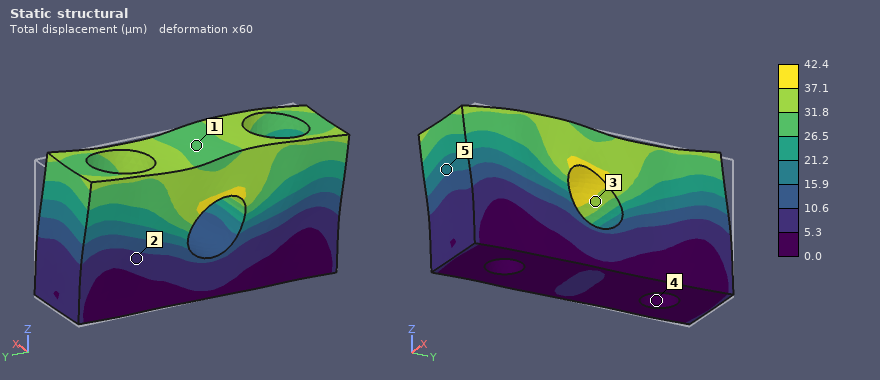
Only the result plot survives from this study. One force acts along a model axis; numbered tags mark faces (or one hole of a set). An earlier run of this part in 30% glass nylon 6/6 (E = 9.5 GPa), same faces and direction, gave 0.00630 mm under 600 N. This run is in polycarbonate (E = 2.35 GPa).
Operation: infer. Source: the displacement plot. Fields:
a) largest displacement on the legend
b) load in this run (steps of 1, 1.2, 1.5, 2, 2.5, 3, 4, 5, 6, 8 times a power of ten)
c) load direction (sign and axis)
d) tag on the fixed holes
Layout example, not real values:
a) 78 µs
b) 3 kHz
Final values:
a) 42.4 µm
b) 1 kN
c) -Y
d) 4
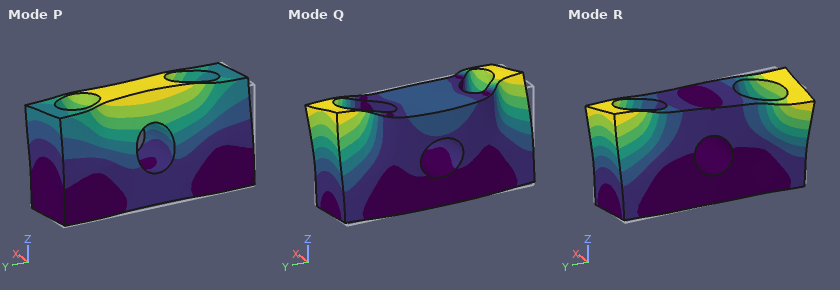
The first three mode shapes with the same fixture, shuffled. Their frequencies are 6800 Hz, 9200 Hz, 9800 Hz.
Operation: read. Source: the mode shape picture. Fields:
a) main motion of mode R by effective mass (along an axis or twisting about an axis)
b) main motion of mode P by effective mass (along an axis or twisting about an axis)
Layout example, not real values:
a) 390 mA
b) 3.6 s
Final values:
a) twisting about Z
b) along X
